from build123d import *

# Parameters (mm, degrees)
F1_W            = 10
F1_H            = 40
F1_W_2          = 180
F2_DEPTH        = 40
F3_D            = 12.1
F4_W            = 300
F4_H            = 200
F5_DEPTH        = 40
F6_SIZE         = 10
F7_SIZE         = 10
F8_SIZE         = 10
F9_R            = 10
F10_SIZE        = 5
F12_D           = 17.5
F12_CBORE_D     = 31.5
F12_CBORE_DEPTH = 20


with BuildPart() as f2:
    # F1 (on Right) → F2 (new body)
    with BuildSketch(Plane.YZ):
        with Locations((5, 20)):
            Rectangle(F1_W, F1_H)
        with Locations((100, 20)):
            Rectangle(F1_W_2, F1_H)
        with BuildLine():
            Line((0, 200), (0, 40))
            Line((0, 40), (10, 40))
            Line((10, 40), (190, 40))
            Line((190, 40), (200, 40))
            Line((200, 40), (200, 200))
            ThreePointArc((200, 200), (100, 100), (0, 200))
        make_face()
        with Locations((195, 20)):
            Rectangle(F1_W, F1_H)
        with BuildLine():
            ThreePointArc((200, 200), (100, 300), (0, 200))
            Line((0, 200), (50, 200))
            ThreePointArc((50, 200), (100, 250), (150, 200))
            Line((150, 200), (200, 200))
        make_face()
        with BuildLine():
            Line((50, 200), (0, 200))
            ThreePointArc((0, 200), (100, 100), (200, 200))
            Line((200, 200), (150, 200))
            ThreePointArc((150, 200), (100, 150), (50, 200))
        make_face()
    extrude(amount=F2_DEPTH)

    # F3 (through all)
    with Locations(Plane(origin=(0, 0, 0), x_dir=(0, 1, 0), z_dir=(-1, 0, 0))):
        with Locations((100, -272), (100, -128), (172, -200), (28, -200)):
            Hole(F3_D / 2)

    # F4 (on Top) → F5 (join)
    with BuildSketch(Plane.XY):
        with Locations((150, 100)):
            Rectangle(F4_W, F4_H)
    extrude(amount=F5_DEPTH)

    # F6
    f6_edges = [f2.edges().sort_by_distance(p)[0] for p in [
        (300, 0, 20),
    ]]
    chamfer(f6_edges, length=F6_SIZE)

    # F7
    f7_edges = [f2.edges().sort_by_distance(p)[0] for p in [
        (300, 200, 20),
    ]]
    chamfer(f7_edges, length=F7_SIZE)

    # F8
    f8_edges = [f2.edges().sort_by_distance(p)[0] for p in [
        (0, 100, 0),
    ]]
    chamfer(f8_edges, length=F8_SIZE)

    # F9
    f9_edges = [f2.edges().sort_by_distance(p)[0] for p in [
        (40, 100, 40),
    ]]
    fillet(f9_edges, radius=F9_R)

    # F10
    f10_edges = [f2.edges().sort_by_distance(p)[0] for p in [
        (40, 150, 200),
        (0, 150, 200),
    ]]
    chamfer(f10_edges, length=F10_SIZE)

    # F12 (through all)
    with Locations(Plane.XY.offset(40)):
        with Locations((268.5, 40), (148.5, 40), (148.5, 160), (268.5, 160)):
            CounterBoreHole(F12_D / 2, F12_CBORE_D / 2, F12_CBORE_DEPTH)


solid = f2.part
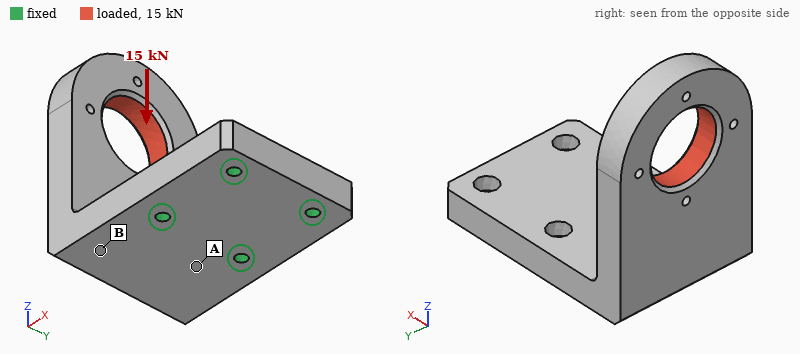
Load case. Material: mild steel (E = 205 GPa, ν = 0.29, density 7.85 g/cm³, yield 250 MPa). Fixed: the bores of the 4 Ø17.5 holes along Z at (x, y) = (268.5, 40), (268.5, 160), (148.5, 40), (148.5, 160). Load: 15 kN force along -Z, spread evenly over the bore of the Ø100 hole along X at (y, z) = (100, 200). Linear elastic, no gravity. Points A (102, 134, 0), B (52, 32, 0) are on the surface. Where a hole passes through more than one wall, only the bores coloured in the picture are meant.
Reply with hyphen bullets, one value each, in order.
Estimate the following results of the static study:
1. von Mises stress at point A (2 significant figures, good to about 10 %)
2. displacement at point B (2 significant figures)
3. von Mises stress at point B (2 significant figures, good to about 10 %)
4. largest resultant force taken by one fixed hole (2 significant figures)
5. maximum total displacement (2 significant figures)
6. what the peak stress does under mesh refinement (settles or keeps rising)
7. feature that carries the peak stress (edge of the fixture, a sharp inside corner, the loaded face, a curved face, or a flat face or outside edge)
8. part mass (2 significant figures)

- 21 MPa
- 0.058 mm
- 8.8 MPa
- 16 kN
- 0.25 mm
- keeps rising
- edge of the fixture
- 30 kg
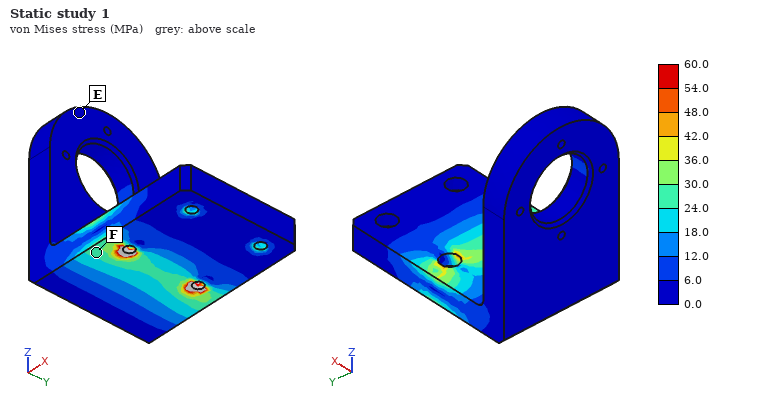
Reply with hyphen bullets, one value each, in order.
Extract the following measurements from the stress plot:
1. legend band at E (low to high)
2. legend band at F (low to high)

- 0.0 to 6.0 MPa
- 24.0 to 30.0 MPa
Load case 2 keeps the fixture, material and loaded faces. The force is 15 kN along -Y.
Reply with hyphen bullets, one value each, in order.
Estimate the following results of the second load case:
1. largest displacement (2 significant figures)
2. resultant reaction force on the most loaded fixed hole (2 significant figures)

- 0.22 mm
- 30 kN
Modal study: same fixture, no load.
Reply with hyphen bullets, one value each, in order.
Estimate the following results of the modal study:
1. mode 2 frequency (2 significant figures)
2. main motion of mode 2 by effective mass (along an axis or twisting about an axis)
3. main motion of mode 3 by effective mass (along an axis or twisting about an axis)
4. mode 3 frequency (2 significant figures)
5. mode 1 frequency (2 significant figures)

- 510 Hz
- along Y
- along Z
- 850 Hz
- 280 Hz
